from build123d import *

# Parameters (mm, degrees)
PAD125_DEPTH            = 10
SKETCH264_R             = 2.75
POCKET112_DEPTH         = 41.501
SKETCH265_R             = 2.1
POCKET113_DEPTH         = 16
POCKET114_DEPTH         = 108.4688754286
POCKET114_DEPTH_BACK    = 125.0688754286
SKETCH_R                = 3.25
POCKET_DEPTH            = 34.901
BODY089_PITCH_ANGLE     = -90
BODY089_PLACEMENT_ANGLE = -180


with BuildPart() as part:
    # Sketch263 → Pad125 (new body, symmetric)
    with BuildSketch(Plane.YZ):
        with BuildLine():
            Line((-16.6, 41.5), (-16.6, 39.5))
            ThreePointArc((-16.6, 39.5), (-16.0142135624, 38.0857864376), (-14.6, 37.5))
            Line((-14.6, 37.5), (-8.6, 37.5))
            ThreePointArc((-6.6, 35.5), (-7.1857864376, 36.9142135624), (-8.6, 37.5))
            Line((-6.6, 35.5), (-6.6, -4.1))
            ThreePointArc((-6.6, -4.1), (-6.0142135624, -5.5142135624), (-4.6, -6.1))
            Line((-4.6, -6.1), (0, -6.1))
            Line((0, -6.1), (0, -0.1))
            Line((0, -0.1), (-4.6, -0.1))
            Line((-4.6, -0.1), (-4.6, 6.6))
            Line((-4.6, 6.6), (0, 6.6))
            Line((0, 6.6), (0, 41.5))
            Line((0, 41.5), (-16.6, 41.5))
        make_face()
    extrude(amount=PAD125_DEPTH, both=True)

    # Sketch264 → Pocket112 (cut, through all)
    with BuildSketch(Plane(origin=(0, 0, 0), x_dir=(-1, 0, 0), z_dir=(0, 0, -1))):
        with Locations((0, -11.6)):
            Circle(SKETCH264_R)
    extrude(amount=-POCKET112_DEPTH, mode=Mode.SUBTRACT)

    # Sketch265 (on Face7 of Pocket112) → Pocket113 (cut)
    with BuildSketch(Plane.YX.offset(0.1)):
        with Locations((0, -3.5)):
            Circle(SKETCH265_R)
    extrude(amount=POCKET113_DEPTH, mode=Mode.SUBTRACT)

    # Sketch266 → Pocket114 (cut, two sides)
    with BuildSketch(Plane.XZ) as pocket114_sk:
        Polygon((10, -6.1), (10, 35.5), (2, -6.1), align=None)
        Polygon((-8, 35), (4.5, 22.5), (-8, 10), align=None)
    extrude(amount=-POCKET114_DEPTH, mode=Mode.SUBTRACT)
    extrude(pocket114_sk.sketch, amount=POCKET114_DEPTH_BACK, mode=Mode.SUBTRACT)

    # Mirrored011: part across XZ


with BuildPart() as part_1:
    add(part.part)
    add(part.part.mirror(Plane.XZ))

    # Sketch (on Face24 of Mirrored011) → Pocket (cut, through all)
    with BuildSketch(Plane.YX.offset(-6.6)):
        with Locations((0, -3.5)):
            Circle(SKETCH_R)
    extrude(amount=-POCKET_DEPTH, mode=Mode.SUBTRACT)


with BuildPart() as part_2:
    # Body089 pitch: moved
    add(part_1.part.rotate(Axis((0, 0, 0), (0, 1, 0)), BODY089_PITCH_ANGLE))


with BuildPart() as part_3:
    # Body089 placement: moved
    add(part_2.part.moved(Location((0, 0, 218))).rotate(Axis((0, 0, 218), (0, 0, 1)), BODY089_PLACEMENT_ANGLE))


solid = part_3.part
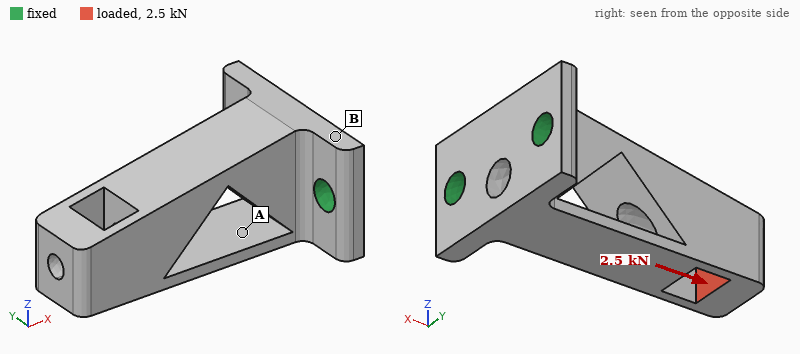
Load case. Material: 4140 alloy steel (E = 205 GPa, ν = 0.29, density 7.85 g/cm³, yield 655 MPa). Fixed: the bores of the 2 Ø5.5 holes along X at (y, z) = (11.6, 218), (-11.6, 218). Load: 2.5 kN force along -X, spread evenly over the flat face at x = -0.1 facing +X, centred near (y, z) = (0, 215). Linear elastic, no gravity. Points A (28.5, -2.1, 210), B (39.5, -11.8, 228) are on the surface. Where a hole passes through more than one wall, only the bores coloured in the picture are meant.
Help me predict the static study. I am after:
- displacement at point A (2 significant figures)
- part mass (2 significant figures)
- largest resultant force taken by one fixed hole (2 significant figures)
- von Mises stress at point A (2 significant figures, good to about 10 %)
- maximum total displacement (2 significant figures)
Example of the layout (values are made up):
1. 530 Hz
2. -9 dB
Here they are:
1. 14 µm
2. 64 g
3. 1.4 kN
4. 57 MPa
5. 44 µm
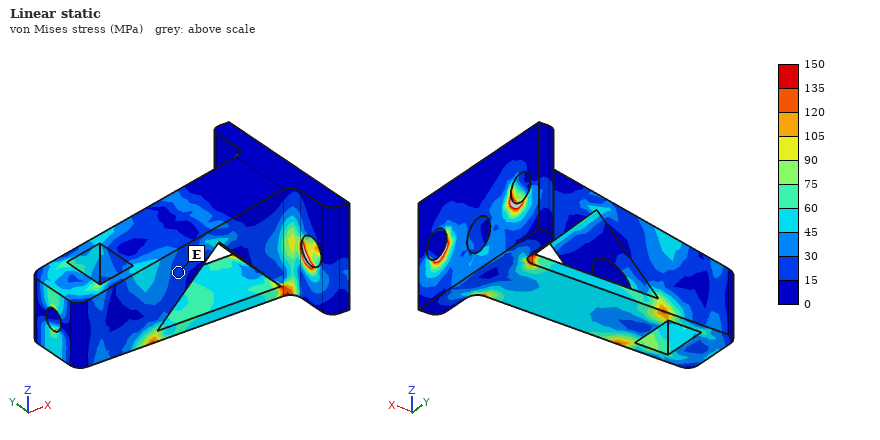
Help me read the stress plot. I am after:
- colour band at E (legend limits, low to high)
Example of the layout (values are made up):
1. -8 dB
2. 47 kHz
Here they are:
1. 15 to 30 MPa
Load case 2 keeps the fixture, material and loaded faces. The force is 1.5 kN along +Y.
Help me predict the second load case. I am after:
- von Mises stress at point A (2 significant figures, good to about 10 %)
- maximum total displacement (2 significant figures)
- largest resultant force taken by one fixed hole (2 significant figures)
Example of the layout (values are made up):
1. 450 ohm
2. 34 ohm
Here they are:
1. 69 MPa
2. 0.18 mm
3. 3.4 kN
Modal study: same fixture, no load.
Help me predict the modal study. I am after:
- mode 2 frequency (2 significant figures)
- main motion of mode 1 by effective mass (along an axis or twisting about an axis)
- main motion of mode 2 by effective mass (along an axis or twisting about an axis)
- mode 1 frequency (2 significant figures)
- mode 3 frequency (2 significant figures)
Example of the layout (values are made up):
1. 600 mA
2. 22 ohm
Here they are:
1. 4200 Hz
2. along Z
3. along Y
4. 3400 Hz
5. 13 kHz
